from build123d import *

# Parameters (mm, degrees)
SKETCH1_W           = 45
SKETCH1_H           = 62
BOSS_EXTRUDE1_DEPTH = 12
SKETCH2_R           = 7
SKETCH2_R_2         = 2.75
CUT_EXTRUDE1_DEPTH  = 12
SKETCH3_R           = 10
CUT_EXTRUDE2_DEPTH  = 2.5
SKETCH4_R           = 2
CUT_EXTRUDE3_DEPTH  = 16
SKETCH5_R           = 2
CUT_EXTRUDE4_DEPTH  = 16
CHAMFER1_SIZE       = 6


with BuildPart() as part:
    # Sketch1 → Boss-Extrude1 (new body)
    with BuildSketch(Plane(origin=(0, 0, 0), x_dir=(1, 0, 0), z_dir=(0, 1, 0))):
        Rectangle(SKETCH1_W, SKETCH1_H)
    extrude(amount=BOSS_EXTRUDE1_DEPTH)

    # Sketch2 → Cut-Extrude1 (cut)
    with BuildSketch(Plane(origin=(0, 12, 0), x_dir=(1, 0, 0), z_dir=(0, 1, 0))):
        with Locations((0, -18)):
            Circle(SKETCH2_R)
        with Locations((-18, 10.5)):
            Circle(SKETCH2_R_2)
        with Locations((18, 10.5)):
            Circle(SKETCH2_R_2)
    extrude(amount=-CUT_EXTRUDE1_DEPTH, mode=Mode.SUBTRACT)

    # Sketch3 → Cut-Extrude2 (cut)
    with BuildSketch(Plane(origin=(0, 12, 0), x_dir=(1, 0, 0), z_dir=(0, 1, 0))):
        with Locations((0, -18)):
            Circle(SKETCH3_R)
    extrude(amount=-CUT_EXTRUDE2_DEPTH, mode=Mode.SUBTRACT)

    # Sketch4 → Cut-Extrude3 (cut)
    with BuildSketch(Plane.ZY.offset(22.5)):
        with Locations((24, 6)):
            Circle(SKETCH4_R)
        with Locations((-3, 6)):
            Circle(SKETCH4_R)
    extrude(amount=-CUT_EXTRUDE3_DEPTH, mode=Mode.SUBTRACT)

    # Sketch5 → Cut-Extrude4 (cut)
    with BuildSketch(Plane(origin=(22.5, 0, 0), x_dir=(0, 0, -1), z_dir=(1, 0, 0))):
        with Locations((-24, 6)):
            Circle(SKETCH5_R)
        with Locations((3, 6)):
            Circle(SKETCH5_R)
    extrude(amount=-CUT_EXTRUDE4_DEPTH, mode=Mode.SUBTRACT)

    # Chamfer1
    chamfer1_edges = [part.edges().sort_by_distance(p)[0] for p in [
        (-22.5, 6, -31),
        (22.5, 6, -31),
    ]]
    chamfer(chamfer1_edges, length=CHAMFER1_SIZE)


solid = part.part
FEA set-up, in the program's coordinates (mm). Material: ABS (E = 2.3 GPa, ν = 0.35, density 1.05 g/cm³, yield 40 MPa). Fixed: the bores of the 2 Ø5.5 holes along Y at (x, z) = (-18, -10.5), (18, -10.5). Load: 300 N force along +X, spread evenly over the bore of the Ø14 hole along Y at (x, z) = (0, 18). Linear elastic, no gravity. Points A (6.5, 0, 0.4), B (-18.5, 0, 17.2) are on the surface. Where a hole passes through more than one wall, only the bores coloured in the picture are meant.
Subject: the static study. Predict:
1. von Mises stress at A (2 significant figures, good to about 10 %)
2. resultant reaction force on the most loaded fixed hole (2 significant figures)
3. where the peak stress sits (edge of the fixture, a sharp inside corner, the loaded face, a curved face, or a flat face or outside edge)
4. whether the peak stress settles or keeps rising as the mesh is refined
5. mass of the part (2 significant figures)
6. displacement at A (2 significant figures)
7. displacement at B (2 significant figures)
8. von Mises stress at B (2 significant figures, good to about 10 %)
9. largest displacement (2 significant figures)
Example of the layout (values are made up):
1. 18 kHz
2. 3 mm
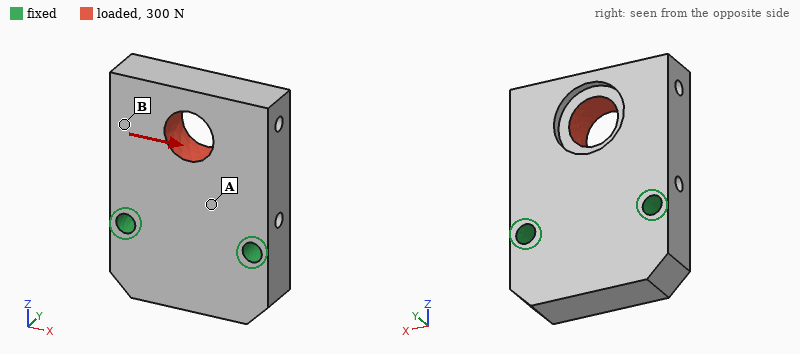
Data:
1. 1.7 MPa
2. 270 N
3. edge of the fixture
4. keeps rising
5. 31 g
6. 12 µm
7. 42 µm
8. 0.77 MPa
9. 65 µm
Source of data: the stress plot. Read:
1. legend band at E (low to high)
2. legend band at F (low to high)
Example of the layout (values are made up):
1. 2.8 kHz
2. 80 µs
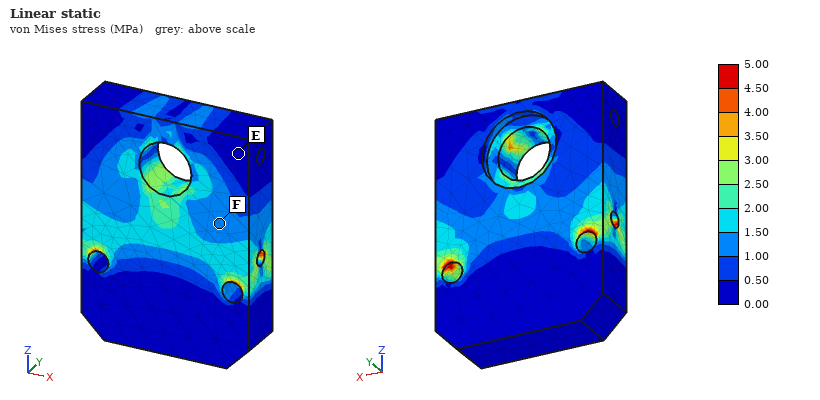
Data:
1. 0.00 to 0.50 MPa
2. 1.00 to 1.50 MPa
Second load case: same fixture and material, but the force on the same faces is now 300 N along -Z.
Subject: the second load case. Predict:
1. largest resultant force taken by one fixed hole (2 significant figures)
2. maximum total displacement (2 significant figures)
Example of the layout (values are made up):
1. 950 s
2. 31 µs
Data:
1. 150 N
2. 34 µm
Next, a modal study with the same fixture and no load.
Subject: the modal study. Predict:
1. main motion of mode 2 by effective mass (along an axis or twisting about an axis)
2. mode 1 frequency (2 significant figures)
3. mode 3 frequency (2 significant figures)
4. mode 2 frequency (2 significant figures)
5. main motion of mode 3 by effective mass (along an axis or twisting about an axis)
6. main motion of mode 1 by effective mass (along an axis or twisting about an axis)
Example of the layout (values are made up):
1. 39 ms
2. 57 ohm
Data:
1. twisting about Z
2. 1500 Hz
3. 3600 Hz
4. 2900 Hz
5. along X
6. along Y
